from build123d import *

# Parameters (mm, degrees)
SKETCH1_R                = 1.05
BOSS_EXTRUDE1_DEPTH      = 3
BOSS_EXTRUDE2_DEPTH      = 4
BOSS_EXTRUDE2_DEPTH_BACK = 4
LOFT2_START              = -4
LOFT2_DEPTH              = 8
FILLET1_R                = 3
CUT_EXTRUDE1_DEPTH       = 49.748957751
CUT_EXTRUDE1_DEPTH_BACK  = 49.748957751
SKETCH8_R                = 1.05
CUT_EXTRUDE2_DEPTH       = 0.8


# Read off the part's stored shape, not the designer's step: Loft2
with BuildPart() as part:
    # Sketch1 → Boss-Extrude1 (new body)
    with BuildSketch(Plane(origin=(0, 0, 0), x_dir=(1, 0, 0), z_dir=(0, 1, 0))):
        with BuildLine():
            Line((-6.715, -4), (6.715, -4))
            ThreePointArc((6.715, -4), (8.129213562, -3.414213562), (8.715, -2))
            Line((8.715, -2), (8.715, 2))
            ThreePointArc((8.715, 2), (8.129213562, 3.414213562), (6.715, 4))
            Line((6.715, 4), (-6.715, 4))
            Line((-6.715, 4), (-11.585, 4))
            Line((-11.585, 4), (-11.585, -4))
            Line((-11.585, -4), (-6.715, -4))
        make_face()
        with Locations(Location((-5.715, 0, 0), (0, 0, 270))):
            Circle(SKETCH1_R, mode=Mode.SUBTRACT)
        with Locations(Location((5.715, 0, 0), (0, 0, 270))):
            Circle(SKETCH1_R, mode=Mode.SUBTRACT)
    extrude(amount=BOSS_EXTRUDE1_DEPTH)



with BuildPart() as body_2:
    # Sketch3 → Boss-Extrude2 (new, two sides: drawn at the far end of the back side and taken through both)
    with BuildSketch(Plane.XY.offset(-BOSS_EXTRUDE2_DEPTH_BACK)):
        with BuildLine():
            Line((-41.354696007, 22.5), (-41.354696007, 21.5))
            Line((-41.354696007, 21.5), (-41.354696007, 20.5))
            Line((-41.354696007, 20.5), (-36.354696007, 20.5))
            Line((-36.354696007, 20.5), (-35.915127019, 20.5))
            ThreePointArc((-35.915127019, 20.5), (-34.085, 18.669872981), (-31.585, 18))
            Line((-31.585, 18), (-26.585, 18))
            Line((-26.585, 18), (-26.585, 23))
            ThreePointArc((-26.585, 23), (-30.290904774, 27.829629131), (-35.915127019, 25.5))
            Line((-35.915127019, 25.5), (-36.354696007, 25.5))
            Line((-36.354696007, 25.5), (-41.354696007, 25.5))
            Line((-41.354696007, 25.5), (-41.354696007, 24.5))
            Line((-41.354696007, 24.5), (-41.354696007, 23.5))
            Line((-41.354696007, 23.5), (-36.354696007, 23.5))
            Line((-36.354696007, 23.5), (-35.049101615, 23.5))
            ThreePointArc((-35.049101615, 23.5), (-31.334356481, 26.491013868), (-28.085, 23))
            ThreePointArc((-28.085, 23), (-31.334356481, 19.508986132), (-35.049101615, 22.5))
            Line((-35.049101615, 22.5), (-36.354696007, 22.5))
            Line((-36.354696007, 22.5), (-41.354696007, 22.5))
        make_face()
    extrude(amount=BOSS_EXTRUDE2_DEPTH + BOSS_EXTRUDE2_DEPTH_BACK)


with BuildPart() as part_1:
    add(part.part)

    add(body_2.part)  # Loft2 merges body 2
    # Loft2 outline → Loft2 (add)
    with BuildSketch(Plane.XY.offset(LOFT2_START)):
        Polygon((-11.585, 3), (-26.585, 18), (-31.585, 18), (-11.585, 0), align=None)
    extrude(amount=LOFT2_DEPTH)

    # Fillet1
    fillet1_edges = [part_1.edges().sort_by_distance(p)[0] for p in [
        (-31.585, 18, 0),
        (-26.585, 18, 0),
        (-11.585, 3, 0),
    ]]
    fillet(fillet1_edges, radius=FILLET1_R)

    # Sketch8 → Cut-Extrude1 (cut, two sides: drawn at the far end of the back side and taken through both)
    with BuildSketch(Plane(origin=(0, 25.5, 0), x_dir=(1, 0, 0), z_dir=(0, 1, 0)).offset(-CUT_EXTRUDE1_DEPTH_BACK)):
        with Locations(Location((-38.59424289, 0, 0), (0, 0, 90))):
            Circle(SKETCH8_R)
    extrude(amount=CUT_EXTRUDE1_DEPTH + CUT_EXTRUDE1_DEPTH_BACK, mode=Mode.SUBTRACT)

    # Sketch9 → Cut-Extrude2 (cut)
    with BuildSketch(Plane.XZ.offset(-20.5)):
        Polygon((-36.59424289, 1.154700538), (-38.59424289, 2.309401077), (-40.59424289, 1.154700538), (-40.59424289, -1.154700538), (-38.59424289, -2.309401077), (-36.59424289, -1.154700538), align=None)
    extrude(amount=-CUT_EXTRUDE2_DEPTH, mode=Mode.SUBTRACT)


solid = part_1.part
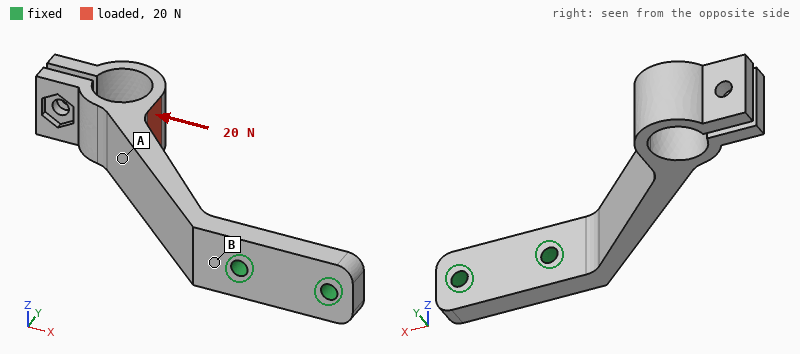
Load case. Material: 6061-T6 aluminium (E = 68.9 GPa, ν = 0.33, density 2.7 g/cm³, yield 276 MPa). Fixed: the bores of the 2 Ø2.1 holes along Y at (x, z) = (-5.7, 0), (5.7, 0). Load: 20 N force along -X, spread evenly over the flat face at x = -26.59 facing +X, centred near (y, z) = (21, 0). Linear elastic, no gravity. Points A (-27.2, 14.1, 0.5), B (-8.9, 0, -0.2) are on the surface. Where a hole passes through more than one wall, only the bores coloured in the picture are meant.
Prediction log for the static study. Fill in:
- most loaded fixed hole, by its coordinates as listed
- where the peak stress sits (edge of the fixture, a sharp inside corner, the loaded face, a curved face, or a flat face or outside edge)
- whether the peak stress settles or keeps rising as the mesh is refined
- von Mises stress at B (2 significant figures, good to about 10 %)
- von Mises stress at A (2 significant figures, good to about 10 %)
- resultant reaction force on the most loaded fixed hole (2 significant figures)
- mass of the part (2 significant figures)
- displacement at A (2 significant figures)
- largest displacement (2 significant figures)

(-5.7, 0)
edge of the fixture
keeps rising
32 MPa
7.7 MPa
19 N
4.0 g
0.12 mm
0.27 mm
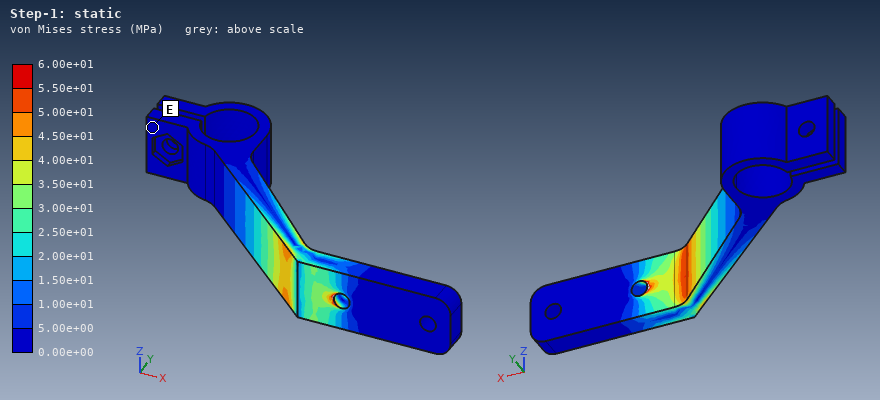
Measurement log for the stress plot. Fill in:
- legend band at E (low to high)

0.00e+00 to 5.00e+00 MPa
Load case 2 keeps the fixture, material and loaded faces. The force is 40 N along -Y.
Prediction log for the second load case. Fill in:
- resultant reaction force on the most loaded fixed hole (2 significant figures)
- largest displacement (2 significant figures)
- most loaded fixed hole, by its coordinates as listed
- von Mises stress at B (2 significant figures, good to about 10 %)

53 N
0.39 mm
(-5.7, 0)
60 MPa
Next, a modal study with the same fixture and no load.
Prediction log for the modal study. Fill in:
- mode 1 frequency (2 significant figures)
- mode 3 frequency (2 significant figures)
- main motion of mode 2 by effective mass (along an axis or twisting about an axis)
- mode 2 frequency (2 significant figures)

960 Hz
4200 Hz
along Z
2100 Hz
